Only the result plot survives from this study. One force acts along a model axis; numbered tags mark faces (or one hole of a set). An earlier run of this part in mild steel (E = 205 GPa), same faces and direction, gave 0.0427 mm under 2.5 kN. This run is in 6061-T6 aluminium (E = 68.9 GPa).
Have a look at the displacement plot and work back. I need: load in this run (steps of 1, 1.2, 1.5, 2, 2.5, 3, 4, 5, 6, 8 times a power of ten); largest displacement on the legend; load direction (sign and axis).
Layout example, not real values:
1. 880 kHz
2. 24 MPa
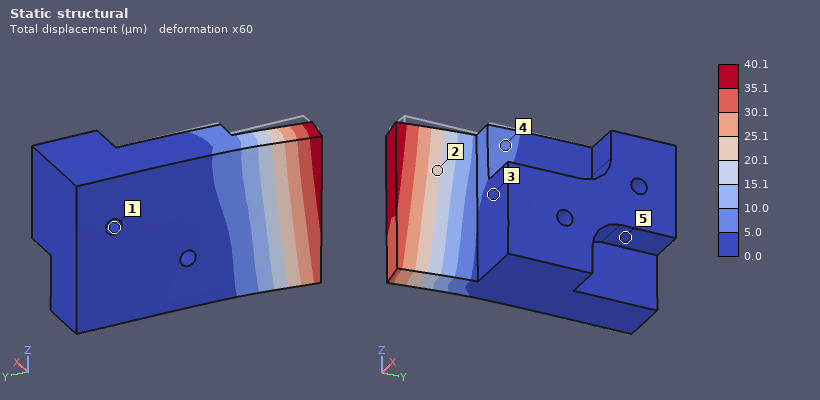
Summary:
1. 800 N
2. 40.1 µm
3. -X
